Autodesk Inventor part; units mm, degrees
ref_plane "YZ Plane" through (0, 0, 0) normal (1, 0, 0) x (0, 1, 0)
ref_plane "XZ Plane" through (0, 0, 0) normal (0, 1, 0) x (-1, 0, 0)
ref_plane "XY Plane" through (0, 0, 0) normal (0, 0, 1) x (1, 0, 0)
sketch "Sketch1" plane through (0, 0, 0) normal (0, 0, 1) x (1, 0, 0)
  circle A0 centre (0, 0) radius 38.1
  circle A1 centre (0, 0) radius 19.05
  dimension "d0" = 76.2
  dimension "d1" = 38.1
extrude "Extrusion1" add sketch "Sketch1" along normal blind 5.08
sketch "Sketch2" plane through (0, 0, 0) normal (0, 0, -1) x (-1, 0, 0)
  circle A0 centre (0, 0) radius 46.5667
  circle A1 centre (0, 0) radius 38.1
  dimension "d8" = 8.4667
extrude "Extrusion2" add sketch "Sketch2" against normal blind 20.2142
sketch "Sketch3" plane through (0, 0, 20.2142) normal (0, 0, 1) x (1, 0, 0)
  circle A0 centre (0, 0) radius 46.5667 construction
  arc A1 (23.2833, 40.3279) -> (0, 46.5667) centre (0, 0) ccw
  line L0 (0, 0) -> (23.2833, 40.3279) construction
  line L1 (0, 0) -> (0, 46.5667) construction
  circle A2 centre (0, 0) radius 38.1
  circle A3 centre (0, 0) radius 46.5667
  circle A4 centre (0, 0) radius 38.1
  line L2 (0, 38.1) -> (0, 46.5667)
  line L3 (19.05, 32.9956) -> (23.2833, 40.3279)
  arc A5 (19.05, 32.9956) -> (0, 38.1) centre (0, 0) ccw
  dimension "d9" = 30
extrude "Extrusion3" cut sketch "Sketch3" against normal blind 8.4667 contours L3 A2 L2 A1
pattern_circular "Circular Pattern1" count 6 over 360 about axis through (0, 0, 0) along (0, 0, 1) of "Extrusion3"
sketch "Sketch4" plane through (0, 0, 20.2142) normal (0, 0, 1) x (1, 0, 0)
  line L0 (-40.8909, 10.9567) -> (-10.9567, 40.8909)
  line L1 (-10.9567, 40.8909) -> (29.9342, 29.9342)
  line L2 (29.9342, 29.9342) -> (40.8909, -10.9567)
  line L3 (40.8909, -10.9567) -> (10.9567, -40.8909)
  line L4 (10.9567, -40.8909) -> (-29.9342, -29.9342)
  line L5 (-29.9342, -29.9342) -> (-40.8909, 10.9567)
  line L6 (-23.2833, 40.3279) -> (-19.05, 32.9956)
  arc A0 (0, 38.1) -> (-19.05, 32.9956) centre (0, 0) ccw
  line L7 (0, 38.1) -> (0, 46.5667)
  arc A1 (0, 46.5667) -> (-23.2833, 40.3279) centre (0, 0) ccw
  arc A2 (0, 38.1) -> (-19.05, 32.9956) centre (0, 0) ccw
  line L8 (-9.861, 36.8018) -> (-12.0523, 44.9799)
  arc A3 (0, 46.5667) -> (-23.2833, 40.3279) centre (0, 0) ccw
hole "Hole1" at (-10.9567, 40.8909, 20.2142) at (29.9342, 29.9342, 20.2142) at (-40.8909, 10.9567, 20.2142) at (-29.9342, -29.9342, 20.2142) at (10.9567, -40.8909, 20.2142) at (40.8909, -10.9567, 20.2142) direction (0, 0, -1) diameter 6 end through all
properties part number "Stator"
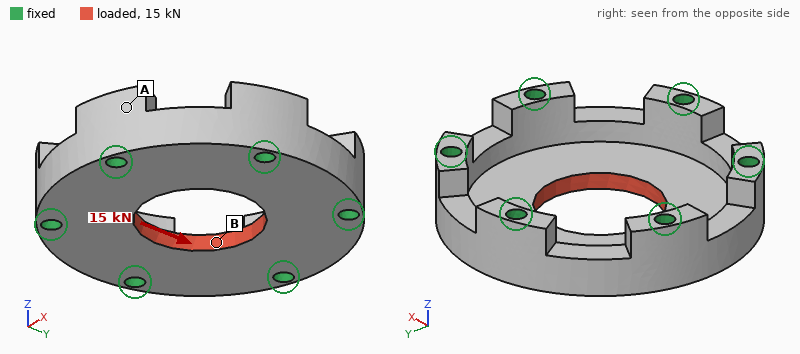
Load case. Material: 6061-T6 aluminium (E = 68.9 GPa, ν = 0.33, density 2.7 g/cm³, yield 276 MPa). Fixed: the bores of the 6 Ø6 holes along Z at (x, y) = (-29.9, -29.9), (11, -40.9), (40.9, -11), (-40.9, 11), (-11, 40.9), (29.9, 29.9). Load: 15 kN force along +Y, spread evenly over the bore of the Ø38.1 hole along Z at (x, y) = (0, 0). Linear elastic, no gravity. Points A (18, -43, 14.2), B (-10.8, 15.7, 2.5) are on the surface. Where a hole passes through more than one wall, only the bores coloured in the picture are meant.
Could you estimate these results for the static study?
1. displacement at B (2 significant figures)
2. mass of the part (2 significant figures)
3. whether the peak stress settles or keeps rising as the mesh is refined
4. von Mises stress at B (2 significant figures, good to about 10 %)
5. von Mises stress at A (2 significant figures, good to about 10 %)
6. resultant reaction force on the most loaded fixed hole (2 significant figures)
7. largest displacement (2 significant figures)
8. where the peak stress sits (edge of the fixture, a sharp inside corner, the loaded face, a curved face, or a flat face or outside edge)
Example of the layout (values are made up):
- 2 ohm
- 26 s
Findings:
- 12 µm
- 130 g
- keeps rising
- 32 MPa
- 7.4 MPa
- 3.3 kN
- 13 µm
- edge of the fixture
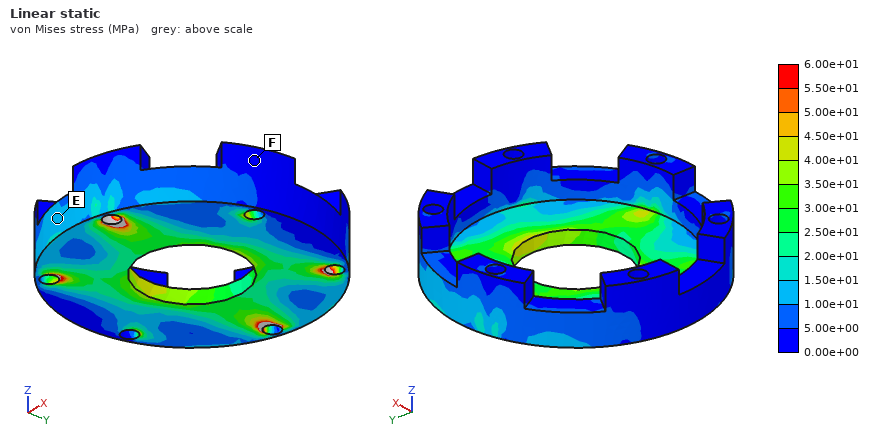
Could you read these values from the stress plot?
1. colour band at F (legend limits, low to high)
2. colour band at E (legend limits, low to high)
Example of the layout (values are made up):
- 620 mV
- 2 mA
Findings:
- 0.00e+00 to 5.00e+00 MPa
- 1.00e+01 to 1.50e+01 MPa
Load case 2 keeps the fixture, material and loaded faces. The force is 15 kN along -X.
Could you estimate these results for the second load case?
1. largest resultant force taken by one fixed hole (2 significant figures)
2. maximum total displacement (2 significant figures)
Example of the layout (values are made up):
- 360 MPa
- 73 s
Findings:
- 3.3 kN
- 13 µm
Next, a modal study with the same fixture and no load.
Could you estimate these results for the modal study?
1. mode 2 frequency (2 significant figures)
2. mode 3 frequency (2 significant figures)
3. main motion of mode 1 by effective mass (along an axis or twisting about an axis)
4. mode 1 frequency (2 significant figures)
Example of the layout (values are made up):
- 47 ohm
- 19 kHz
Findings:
- 14 kHz
- 14 kHz
- along Z
- 11 kHz
